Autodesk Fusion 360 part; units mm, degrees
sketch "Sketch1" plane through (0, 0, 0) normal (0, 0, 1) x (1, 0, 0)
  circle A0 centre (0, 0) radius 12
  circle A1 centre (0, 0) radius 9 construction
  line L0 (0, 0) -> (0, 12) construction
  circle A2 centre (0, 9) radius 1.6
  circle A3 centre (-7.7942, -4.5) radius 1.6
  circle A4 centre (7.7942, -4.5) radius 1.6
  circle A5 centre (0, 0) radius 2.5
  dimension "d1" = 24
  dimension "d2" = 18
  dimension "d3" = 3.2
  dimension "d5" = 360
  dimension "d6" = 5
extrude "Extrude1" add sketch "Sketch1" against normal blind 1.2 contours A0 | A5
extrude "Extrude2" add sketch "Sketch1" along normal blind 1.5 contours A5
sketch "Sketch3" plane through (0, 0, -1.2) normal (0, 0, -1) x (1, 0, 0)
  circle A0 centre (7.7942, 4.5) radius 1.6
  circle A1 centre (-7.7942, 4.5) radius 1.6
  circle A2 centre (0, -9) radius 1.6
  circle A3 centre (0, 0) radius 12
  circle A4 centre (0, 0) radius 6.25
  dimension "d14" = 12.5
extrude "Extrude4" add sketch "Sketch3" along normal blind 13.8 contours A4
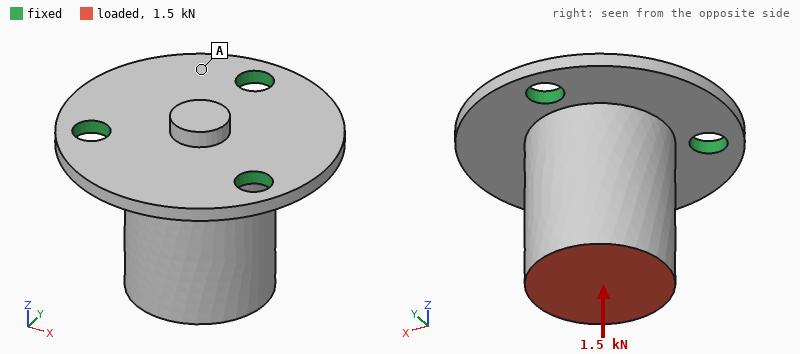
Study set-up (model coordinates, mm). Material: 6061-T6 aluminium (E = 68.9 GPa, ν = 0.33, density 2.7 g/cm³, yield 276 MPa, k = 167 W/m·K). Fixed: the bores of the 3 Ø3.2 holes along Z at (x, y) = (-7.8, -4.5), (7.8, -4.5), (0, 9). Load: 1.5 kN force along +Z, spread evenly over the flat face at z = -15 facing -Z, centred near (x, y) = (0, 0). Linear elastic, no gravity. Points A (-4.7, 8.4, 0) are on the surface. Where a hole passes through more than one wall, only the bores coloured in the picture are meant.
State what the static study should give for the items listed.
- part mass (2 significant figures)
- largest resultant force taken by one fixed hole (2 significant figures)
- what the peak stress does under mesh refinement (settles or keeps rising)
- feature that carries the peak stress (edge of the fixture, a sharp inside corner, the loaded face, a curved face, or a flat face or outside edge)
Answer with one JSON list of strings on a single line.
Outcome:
["6.0 g", "550 N", "keeps rising", "edge of the fixture"]
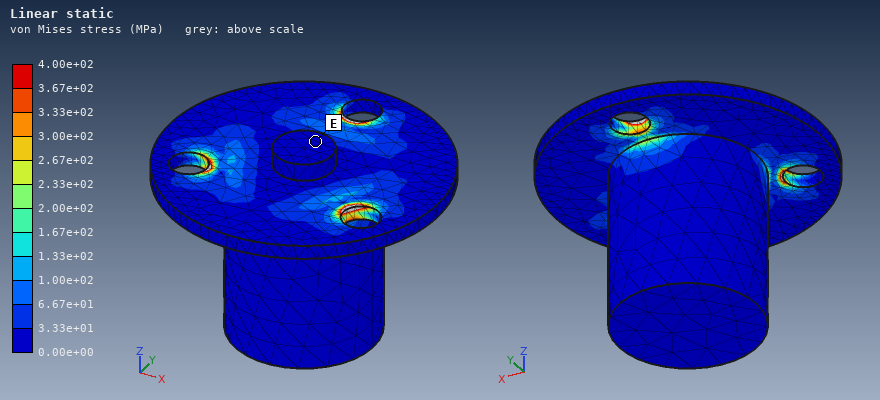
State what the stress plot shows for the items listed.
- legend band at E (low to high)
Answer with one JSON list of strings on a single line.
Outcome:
["0.00e+00 to 3.33e+01 MPa"]
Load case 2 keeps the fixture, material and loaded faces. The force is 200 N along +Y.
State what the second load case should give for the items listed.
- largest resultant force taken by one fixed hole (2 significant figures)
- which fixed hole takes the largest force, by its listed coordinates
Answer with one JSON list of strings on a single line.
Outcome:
["290 N", "(0, 9)"]
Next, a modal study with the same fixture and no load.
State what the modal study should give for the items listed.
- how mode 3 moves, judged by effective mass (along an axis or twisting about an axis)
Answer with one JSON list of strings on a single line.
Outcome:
["along Z"]
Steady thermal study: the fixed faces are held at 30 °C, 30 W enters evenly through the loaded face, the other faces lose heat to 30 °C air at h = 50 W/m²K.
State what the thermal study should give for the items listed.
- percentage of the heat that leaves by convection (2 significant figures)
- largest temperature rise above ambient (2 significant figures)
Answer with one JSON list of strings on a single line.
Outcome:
["3.6 %", "36 K"]
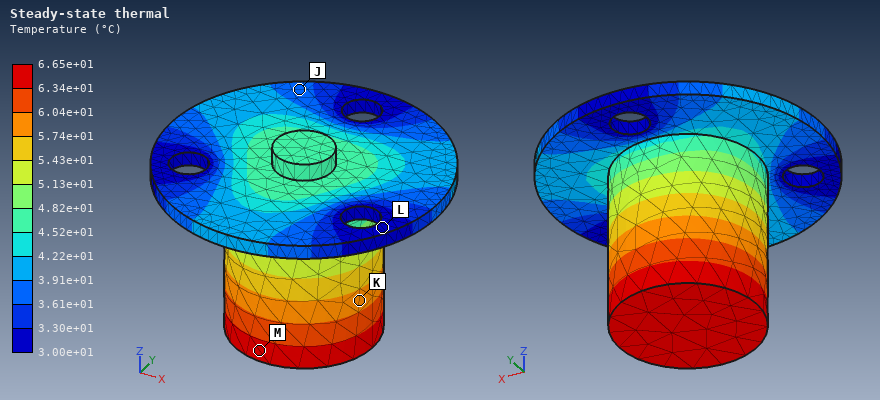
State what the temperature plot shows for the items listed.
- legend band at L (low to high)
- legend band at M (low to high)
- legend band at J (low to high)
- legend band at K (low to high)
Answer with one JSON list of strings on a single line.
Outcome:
["3.00e+01 to 3.30e+01 °C", "6.34e+01 to 6.65e+01 °C", "3.61e+01 to 3.91e+01 °C", "5.74e+01 to 6.04e+01 °C"]
